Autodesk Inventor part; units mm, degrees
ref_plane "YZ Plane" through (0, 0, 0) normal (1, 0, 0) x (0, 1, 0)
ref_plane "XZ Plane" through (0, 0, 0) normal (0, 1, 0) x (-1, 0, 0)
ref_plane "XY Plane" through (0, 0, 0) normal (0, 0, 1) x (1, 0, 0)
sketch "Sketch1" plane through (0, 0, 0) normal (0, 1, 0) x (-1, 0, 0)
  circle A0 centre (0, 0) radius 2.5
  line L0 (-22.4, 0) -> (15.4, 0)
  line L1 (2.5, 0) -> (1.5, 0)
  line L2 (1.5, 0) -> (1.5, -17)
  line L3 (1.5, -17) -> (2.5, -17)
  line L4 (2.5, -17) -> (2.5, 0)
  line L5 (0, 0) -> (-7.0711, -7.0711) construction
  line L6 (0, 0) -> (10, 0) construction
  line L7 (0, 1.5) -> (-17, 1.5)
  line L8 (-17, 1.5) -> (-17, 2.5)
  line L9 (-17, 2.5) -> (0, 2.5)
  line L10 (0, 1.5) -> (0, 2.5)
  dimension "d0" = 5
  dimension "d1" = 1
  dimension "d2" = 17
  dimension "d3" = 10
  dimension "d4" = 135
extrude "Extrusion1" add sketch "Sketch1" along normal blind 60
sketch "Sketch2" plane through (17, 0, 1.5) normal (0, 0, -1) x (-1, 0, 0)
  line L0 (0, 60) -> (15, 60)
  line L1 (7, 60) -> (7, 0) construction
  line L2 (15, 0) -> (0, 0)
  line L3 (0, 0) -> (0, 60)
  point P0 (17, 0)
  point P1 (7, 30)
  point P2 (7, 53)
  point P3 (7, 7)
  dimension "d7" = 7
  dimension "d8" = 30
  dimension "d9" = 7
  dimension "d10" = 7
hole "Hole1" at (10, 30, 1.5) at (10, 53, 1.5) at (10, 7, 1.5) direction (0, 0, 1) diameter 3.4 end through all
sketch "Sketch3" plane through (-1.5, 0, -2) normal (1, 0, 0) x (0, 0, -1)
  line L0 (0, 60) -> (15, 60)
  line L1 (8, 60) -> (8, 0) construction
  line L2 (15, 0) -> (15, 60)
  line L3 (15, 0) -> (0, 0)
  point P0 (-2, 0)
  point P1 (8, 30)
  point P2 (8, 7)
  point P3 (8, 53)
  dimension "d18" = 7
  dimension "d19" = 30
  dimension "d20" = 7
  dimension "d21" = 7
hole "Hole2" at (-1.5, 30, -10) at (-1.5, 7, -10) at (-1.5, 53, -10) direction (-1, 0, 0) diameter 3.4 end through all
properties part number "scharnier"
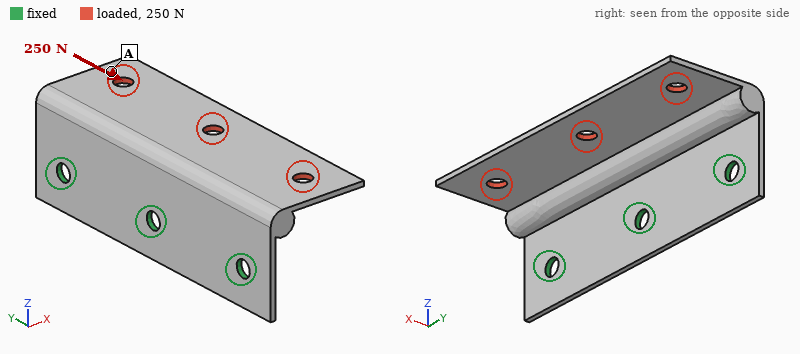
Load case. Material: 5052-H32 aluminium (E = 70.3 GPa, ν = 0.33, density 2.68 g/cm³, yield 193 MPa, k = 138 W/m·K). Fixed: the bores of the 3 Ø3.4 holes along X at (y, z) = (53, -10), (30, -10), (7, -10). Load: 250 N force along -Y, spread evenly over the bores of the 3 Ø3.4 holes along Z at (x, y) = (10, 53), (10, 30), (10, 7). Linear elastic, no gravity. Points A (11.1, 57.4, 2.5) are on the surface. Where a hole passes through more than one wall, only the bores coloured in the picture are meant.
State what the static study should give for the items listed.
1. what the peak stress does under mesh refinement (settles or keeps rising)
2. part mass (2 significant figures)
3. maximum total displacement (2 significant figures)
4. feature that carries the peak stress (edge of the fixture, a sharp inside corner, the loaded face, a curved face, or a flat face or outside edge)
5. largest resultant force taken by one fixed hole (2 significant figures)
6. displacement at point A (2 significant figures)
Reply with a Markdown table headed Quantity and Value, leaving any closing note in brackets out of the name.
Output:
| Quantity | Value |
|---|---|
| what the peak stress does under mesh refinement | keeps rising |
| part mass | 8.0 g |
| maximum total displacement | 0.11 mm |
| feature that carries the peak stress | edge of the fixture |
| largest resultant force taken by one fixed hole | 110 N |
| displacement at point A | 0.091 mm |
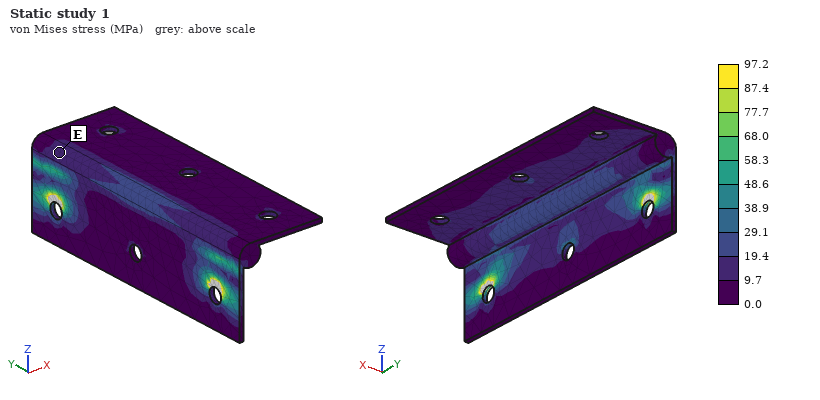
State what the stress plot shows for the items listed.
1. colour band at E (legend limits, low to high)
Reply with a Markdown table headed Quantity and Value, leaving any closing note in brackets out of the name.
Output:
| Quantity | Value |
|---|---|
| colour band at E | 9.7 to 19.4 MPa |
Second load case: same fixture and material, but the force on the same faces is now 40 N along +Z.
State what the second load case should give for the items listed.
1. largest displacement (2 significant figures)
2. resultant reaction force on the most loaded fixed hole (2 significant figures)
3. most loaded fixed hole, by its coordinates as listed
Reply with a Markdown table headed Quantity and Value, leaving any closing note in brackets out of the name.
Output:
| Quantity | Value |
|---|---|
| largest displacement | 0.27 mm |
| resultant reaction force on the most loaded fixed hole | 18 N |
| most loaded fixed hole, by its coordinates as listed | (30, -10) |
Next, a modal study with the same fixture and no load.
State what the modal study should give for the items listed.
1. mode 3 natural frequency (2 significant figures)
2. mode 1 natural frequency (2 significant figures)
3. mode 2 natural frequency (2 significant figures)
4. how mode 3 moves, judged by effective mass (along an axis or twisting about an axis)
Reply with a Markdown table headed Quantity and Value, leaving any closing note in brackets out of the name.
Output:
| Quantity | Value |
|---|---|
| mode 3 natural frequency | 4300 Hz |
| mode 1 natural frequency | 1300 Hz |
| mode 2 natural frequency | 3100 Hz |
| how mode 3 moves, judged by effective mass | along X |
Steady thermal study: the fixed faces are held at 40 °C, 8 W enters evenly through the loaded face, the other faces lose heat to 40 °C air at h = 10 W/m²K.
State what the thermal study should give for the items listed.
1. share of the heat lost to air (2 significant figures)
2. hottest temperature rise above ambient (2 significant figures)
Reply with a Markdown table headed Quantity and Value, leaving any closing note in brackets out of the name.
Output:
| Quantity | Value |
|---|---|
| share of the heat lost to air | 6.0 % |
| hottest temperature rise above ambient | 23 K |
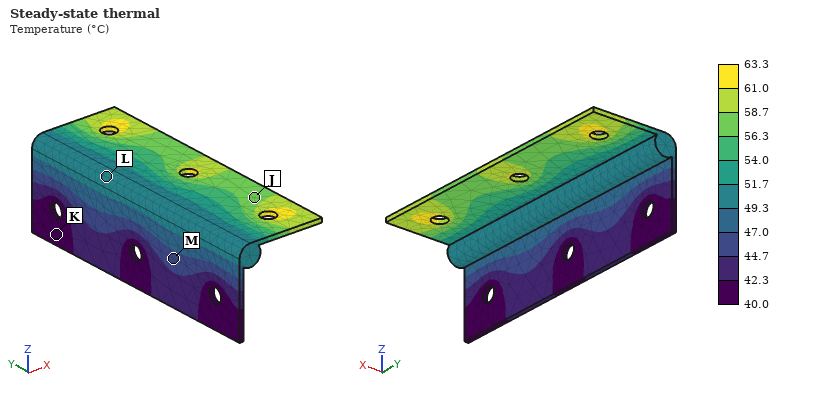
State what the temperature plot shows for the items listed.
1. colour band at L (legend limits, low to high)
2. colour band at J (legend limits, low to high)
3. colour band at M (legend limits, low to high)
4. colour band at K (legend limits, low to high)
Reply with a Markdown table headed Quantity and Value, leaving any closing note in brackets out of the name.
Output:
| Quantity | Value |
|---|---|
| colour band at L | 49.3 to 51.7 °C |
| colour band at J | 56.3 to 58.7 °C |
| colour band at M | 44.7 to 47.0 °C |
| colour band at K | 40.0 to 42.3 °C |
